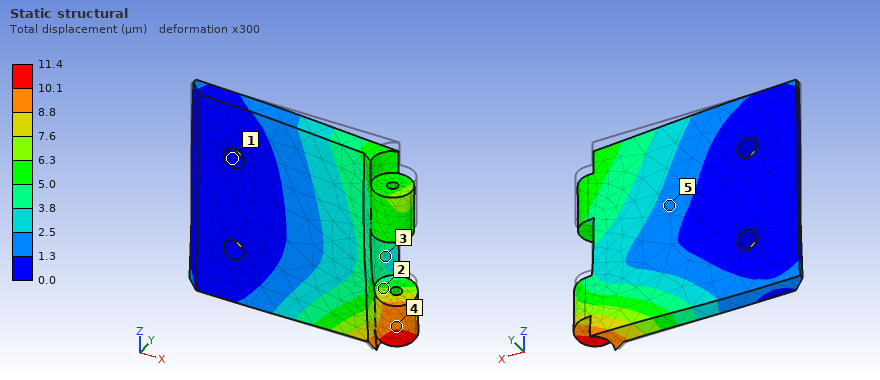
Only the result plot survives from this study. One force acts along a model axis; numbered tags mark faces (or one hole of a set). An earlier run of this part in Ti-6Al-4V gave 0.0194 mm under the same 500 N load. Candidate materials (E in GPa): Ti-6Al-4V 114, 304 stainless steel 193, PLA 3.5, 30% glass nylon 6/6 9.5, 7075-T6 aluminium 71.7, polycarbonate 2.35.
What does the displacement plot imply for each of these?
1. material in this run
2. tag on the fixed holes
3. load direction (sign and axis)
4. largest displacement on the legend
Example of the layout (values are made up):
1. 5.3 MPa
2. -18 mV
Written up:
1. 304 stainless steel
2. 1
3. -Z
4. 11.4 µm
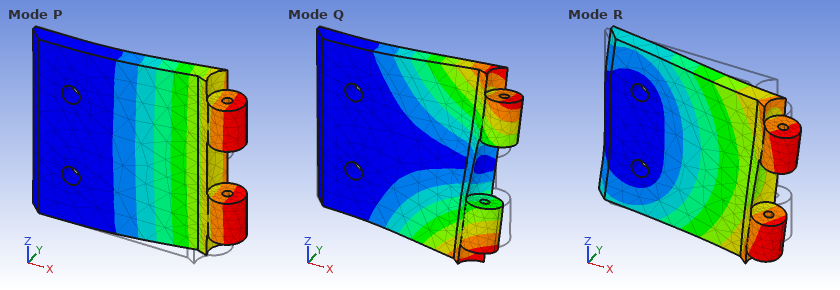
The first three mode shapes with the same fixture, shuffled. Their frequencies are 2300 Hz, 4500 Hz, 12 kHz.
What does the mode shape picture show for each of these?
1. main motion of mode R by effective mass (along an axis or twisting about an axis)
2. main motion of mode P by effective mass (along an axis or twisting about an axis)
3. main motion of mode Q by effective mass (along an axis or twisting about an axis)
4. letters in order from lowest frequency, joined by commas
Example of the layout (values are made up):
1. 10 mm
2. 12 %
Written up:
1. along Z
2. along Y
3. twisting about X
4. P, Q, R
